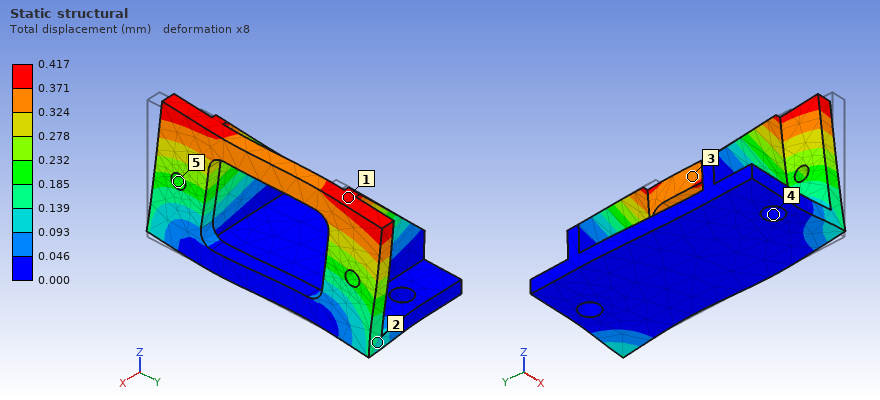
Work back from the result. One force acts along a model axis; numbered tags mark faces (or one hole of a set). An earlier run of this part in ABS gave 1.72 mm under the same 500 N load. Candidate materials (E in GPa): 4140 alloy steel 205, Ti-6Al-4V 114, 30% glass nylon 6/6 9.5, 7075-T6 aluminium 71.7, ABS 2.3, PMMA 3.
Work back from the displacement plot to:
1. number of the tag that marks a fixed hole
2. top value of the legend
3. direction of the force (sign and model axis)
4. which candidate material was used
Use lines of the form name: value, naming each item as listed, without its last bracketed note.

number of the tag that marks a fixed hole: 4
top value of the legend: 0.417 mm
direction of the force: +Y
which candidate material was used: 30% glass nylon 6/6
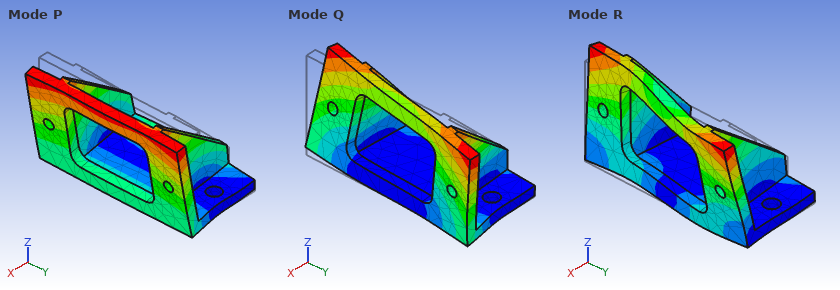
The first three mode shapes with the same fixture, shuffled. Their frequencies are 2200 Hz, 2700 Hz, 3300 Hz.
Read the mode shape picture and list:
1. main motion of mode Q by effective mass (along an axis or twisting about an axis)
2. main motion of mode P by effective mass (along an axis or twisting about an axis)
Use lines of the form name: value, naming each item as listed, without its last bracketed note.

main motion of mode Q by effective mass: along Y
main motion of mode P by effective mass: along X
